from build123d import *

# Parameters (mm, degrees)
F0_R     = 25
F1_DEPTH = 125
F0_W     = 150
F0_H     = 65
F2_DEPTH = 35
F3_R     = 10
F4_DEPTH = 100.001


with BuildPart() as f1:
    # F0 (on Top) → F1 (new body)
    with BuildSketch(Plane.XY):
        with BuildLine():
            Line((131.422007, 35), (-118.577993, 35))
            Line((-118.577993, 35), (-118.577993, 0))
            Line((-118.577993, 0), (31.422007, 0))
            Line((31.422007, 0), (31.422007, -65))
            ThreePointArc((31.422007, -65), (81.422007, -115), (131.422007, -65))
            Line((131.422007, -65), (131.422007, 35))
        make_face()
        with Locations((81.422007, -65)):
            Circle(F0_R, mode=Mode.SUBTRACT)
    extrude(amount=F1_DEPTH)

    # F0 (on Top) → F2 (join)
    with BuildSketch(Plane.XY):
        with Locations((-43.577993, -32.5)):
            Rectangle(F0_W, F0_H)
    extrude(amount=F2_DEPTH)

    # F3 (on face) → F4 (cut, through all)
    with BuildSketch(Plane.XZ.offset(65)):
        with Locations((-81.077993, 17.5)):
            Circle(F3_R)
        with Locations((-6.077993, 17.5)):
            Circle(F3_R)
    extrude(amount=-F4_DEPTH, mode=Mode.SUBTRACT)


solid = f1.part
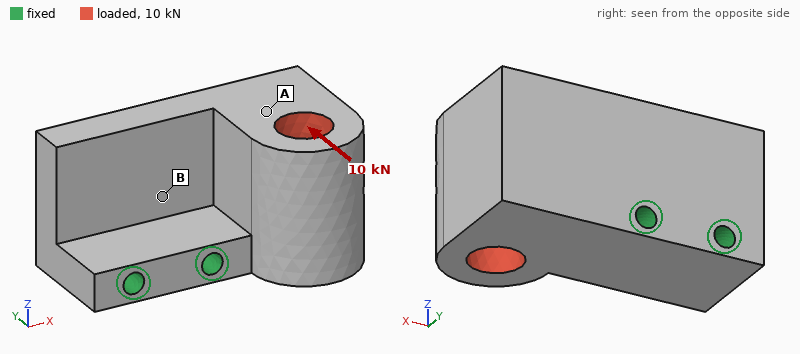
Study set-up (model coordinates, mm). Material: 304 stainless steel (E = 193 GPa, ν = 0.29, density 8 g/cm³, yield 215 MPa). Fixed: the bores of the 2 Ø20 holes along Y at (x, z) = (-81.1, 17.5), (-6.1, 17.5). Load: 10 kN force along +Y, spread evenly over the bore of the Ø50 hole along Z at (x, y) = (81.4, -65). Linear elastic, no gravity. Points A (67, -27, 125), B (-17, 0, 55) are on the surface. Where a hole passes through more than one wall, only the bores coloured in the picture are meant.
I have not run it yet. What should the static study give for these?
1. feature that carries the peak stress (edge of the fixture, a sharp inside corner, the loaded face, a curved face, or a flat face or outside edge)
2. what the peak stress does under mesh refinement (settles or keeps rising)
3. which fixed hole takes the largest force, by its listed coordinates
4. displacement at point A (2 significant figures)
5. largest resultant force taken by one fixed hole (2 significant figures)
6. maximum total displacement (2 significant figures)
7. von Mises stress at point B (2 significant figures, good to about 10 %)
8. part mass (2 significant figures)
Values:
edge of the fixture
keeps rising
(-6.1, 17.5)
11 µm
10 kN
16 µm
3.5 MPa
19 kg
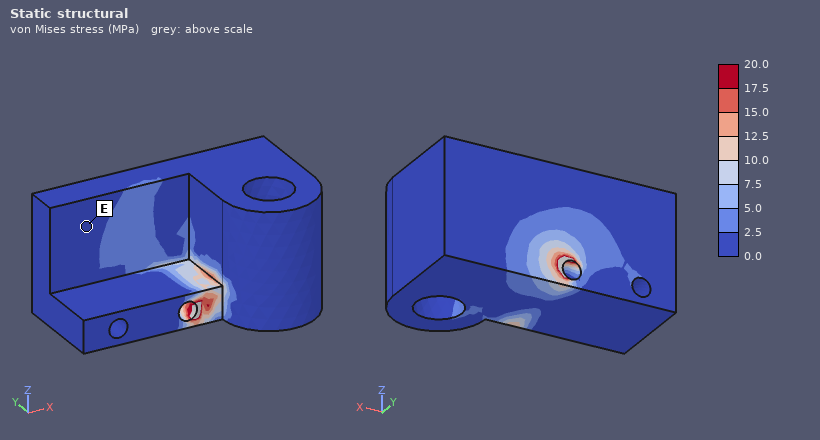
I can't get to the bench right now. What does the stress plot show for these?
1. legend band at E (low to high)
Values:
0.0 to 2.5 MPa
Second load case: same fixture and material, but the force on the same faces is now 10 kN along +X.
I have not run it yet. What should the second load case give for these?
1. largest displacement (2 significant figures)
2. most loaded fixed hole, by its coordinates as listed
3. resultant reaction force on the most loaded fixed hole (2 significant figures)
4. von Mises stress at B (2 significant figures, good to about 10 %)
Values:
17 µm
(-6.1, 17.5)
8.7 kN
3.7 MPa
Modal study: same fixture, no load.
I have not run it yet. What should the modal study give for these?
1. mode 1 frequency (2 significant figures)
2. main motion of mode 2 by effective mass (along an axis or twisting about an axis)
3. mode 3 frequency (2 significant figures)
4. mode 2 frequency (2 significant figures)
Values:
1300 Hz
along Y
2300 Hz
1400 Hz
